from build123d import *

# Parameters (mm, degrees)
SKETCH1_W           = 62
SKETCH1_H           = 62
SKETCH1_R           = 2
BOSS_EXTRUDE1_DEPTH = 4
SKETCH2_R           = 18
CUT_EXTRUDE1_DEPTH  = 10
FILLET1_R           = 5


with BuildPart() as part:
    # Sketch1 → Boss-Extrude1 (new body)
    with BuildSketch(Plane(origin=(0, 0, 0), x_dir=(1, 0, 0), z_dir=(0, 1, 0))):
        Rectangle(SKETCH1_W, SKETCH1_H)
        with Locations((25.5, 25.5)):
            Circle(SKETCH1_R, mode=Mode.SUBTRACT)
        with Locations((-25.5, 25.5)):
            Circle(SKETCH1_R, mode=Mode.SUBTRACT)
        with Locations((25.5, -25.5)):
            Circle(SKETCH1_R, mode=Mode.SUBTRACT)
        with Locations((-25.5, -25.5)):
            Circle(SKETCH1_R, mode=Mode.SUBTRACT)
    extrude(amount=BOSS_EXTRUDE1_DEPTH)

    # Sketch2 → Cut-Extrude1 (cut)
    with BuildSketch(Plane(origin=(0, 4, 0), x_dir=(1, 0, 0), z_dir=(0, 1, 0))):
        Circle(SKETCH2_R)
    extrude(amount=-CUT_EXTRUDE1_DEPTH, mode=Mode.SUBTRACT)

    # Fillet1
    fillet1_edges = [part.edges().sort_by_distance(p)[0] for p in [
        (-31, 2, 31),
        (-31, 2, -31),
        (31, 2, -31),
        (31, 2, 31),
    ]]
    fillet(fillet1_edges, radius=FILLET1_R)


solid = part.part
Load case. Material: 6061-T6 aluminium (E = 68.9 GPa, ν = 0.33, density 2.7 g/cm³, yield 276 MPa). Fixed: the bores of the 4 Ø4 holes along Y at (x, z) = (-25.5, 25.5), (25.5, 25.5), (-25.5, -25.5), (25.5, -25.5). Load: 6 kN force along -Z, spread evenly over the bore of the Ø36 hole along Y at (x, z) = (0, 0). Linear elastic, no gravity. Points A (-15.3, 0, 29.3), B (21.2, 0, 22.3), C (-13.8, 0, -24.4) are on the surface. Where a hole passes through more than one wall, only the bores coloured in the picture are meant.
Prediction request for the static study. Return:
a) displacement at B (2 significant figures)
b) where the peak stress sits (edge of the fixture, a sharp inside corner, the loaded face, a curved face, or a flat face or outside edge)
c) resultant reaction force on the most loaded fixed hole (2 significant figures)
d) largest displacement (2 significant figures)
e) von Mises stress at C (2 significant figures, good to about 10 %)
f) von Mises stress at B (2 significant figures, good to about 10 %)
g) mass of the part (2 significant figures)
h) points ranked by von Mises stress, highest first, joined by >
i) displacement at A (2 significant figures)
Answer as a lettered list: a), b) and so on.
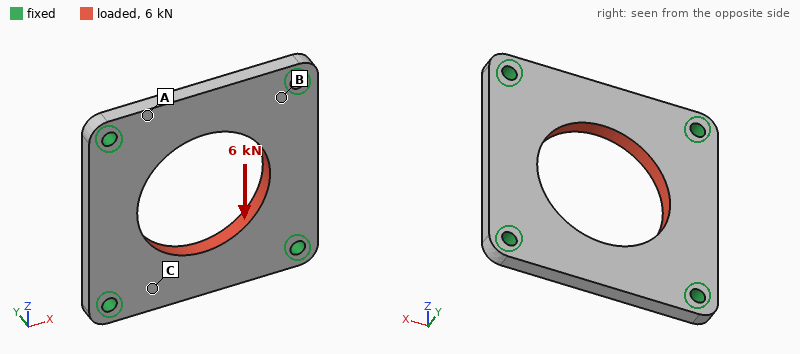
a) 4.0 µm
b) edge of the fixture
c) 1.6 kN
d) 19 µm
e) 19 MPa
f) 30 MPa
g) 30 g
h) B > C > A
i) 9.8 µm
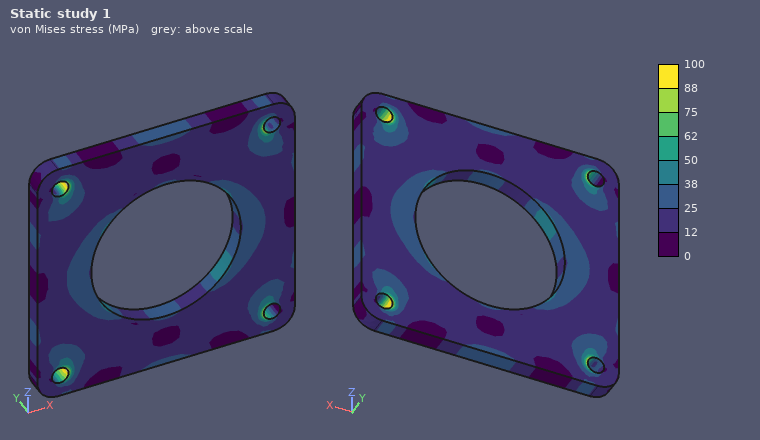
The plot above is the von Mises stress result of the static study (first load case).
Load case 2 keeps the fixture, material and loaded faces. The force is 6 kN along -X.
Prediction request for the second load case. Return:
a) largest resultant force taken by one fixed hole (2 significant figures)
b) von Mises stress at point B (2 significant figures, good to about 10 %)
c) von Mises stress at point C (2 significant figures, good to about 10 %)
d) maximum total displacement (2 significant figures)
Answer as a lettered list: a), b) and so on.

a) 1.6 kN
b) 33 MPa
c) 20 MPa
d) 19 µm
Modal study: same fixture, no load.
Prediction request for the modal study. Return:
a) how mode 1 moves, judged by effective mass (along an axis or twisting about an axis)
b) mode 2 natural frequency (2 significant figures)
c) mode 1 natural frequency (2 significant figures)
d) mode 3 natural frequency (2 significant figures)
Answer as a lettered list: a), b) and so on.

a) along Y
b) 8500 Hz
c) 7300 Hz
d) 8500 Hz
